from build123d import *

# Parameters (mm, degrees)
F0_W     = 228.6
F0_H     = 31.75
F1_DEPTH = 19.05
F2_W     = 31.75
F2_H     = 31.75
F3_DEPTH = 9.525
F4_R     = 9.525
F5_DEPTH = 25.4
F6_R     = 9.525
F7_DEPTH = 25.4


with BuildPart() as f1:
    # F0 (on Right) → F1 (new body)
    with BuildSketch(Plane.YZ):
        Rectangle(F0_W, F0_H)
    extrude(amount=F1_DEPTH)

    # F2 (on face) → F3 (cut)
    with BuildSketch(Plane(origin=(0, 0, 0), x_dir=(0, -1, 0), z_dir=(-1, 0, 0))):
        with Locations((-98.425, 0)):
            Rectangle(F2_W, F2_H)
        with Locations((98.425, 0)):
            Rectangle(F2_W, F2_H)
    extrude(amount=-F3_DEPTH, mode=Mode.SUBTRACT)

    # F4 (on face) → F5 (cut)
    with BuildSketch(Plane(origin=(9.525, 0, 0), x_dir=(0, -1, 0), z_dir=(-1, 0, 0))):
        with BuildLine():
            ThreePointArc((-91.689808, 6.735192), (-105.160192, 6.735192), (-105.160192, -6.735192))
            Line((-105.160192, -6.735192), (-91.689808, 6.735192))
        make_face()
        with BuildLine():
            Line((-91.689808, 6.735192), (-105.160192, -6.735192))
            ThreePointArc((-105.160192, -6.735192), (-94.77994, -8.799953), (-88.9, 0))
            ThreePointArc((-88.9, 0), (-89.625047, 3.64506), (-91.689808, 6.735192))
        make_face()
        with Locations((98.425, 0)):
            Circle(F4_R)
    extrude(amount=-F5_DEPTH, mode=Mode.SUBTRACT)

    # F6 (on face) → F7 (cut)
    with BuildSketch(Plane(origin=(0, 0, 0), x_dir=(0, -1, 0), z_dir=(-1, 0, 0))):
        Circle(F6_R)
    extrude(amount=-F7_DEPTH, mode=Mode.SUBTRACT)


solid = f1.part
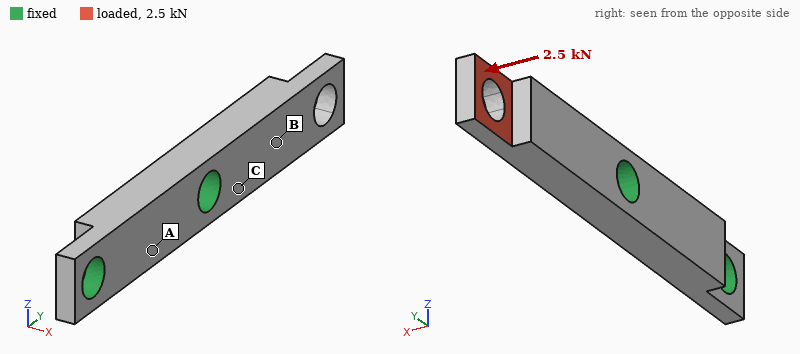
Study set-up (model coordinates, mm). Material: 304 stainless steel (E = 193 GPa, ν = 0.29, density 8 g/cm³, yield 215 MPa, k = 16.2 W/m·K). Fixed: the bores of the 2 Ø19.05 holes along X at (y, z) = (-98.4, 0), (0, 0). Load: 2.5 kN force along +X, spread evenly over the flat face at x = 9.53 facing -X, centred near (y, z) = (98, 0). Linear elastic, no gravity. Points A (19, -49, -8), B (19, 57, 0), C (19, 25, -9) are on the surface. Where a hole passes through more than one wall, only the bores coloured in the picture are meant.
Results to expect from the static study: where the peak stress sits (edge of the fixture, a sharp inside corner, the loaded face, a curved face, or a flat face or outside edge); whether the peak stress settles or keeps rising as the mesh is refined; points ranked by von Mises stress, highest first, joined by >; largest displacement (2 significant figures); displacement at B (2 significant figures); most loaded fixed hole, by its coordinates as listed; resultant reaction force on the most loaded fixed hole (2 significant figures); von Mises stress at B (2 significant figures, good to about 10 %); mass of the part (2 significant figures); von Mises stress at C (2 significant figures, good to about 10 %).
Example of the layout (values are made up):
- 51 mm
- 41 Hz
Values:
- edge of the fixture
- keeps rising
- C > B > A
- 0.29 mm
- 0.074 mm
- (0, 0)
- 2.5 kN
- 54 MPa
- 870 g
- 95 MPa
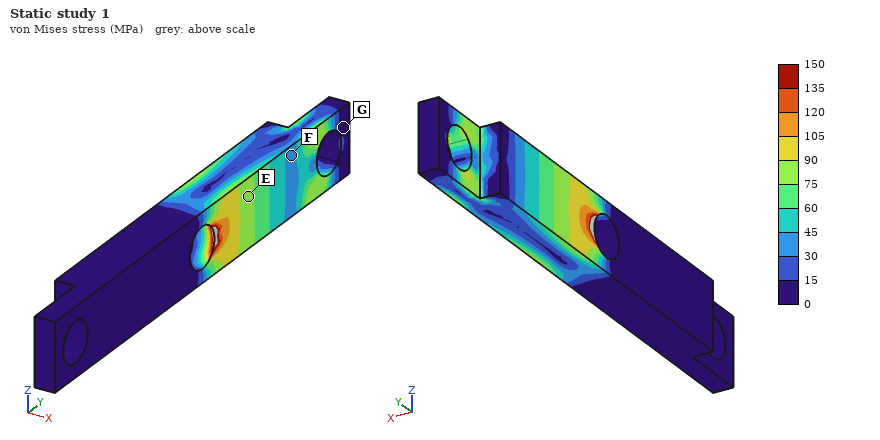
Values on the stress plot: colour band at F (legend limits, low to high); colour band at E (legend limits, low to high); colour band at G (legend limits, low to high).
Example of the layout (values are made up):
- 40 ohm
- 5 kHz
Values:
- 30 to 45 MPa
- 75 to 90 MPa
- 0 to 15 MPa
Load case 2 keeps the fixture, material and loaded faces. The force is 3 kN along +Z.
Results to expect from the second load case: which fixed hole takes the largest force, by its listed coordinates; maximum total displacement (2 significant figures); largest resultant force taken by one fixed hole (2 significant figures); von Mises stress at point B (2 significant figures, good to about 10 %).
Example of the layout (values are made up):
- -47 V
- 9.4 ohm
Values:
- (0, 0)
- 0.15 mm
- 3.2 kN
- 11 MPa
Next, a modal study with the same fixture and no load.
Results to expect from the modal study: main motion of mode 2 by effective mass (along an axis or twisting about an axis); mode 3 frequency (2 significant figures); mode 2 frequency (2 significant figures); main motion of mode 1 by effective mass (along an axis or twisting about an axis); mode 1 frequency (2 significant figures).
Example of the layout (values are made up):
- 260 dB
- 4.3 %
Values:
- along Z
- 5800 Hz
- 2500 Hz
- along X
- 1700 Hz
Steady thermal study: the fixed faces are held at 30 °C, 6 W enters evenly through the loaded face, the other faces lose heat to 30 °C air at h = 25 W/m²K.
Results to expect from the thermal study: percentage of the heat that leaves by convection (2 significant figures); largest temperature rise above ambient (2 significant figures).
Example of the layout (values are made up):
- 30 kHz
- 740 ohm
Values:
- 65 %
- 45 K
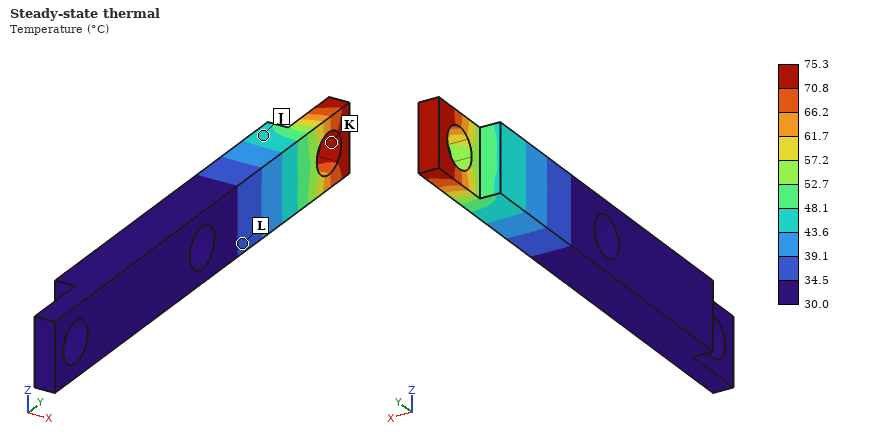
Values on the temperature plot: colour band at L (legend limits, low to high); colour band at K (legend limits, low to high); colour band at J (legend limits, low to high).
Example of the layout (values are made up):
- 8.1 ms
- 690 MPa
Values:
- 34.5 to 39.1 °C
- 70.8 to 75.3 °C
- 43.6 to 48.1 °C
